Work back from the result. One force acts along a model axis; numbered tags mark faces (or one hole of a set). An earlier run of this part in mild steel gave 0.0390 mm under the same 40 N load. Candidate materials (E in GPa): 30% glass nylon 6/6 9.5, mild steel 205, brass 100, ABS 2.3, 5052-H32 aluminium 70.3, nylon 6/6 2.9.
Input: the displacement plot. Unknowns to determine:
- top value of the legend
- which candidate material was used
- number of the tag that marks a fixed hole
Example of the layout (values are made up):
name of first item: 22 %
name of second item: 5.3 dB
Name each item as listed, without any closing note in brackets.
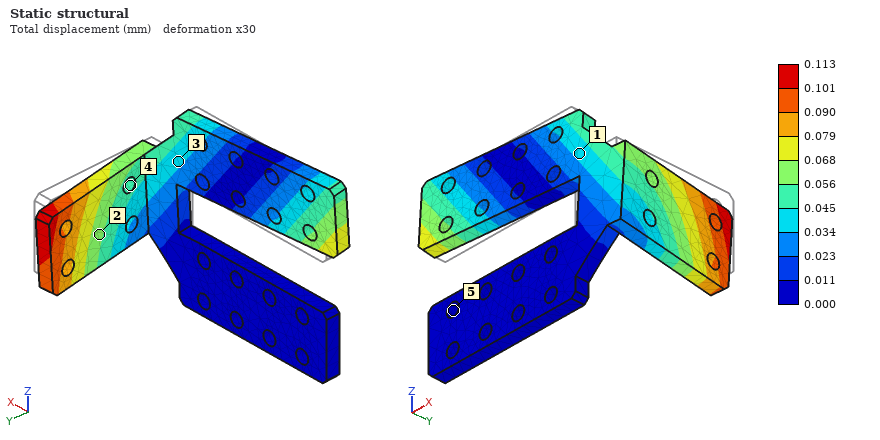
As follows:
top value of the legend: 0.113 mm
which candidate material was used: 5052-H32 aluminium
number of the tag that marks a fixed hole: 5
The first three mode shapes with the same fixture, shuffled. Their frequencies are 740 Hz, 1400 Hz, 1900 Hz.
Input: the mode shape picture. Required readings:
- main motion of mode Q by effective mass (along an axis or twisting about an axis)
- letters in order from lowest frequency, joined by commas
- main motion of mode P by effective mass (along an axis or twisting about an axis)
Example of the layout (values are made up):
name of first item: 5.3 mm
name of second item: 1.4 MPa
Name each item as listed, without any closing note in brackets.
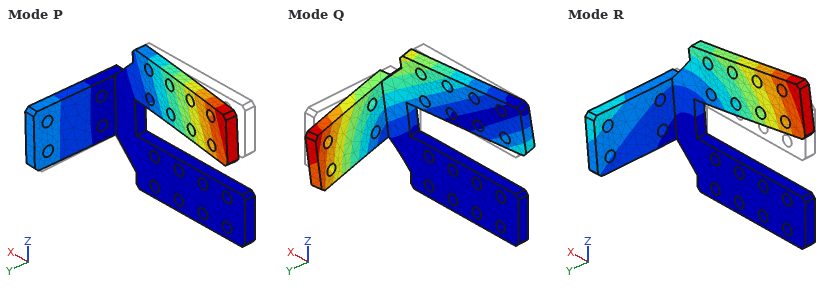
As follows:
main motion of mode Q by effective mass: along Y
letters in order from lowest frequency, joined by commas: P, Q, R
main motion of mode P by effective mass: along Y
